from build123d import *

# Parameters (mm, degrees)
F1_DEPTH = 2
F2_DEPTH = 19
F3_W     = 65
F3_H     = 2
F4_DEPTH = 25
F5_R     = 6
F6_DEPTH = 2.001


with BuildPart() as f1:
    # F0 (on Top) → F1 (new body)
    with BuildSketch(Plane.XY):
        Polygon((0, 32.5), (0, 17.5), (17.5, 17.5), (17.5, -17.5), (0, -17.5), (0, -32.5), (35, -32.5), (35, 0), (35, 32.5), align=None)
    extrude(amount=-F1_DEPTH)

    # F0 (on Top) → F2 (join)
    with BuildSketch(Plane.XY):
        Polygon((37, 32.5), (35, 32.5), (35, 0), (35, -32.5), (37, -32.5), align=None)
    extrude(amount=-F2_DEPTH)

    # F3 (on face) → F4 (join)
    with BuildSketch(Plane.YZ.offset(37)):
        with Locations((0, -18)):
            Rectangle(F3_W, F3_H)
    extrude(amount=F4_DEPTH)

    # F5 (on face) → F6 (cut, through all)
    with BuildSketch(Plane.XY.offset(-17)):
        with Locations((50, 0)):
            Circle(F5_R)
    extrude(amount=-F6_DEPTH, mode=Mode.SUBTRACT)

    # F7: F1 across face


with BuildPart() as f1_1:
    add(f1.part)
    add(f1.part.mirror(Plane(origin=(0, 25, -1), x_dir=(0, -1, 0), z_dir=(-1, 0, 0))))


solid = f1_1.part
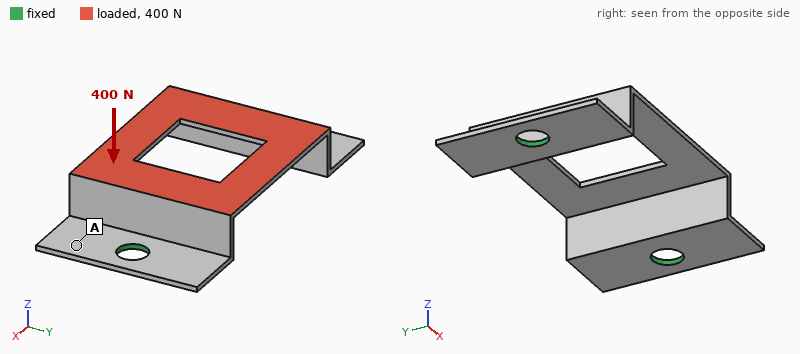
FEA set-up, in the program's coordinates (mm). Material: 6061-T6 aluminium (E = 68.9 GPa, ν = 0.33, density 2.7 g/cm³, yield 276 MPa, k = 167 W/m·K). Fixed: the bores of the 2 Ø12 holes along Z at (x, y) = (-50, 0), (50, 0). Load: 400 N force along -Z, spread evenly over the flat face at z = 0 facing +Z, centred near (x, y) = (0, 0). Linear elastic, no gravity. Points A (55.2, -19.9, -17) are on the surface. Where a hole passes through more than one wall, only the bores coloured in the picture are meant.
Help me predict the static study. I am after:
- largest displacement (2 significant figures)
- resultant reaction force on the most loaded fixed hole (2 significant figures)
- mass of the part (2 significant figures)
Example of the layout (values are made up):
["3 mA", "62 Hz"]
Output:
["0.20 mm", "280 N", "48 g"]
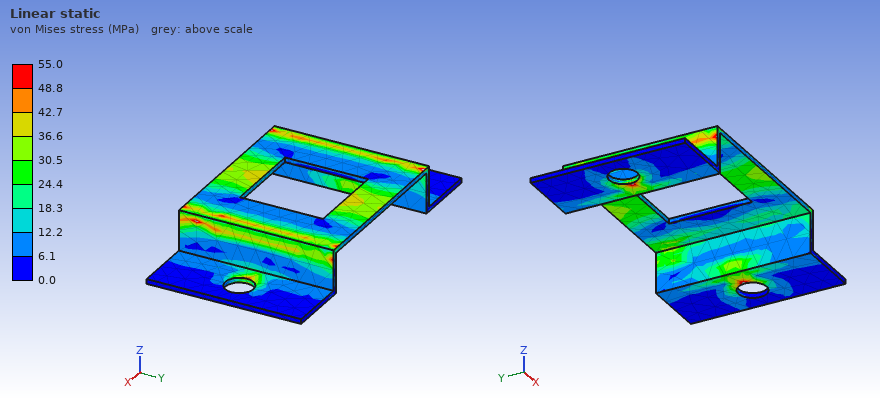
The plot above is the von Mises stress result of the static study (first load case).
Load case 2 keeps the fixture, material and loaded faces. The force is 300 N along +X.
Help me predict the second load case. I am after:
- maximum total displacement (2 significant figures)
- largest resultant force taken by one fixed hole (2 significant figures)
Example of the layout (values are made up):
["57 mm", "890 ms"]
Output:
["0.14 mm", "150 N"]
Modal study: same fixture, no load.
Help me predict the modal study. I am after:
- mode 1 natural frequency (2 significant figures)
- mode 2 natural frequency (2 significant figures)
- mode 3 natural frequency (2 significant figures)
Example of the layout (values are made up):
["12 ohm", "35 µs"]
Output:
["1200 Hz", "1600 Hz", "1600 Hz"]
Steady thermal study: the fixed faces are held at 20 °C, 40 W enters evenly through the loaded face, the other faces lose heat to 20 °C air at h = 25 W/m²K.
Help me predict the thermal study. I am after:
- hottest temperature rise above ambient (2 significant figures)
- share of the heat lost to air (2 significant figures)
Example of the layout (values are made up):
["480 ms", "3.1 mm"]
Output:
["43 K", "18 %"]
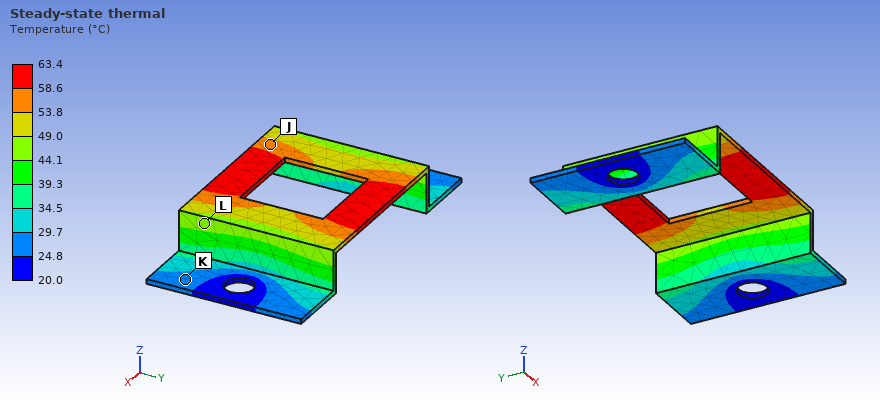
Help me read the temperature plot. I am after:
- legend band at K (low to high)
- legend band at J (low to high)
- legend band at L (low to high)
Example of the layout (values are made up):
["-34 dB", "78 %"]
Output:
["24.8 to 29.7 °C", "53.8 to 58.6 °C", "44.1 to 49.0 °C"]
